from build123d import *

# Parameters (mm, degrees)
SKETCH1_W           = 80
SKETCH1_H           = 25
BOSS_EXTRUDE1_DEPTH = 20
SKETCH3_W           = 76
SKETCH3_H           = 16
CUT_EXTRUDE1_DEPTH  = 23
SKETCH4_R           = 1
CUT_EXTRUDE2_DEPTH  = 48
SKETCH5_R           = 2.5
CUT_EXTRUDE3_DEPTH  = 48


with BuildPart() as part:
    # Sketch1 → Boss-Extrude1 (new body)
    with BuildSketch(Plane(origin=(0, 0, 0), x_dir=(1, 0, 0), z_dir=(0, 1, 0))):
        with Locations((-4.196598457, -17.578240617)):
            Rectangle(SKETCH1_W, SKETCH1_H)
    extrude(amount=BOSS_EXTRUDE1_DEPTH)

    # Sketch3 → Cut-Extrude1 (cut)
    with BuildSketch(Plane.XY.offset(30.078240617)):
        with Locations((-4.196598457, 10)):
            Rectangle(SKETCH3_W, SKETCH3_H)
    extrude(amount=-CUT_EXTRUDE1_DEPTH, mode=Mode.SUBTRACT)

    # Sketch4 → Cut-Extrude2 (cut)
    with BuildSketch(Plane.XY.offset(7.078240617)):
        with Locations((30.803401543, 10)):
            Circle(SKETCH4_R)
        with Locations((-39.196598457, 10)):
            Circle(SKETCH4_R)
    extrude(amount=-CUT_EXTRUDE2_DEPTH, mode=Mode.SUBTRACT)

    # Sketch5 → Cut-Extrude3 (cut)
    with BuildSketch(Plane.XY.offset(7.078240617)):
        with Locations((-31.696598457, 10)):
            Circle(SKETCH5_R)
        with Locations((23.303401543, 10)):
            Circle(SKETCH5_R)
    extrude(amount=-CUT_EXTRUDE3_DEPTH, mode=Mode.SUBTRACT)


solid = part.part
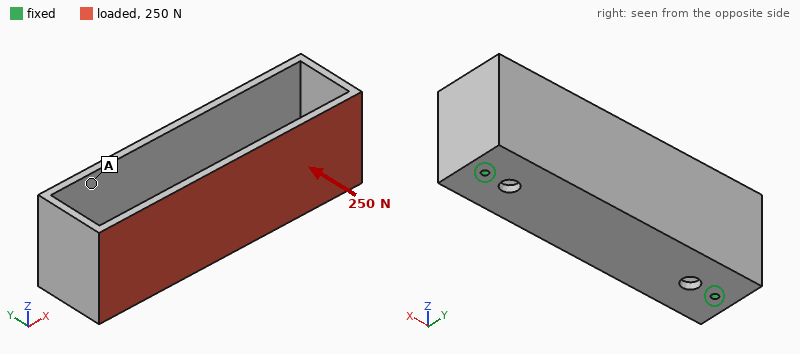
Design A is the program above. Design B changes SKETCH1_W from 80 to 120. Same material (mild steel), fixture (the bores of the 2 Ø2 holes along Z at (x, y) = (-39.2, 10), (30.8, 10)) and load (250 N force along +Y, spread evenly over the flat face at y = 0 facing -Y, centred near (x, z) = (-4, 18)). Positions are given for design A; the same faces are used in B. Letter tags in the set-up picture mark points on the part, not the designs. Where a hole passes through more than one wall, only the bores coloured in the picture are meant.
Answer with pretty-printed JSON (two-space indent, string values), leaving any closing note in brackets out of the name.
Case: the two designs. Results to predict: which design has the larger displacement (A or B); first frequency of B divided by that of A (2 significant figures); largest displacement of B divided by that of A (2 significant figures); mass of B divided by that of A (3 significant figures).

{
  "which design has the larger displacement": "A",
  "first frequency of B divided by that of A": "0.64",
  "largest displacement of B divided by that of A": "0.77",
  "mass of B divided by that of A": "2.67"
}
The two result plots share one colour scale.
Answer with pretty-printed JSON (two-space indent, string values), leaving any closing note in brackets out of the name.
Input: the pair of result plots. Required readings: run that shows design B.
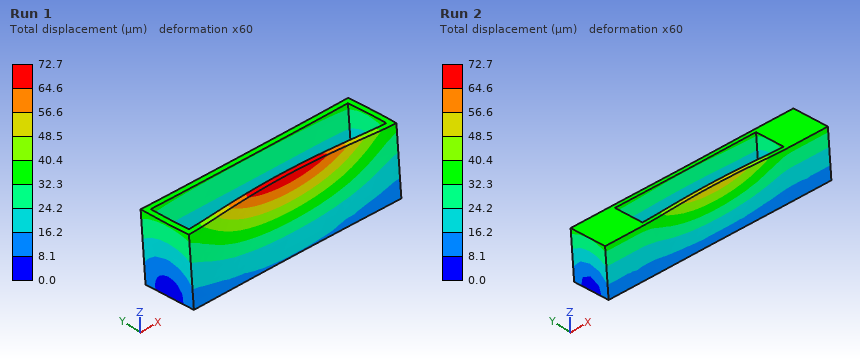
{
  "run that shows design B": "Run 2"
}
